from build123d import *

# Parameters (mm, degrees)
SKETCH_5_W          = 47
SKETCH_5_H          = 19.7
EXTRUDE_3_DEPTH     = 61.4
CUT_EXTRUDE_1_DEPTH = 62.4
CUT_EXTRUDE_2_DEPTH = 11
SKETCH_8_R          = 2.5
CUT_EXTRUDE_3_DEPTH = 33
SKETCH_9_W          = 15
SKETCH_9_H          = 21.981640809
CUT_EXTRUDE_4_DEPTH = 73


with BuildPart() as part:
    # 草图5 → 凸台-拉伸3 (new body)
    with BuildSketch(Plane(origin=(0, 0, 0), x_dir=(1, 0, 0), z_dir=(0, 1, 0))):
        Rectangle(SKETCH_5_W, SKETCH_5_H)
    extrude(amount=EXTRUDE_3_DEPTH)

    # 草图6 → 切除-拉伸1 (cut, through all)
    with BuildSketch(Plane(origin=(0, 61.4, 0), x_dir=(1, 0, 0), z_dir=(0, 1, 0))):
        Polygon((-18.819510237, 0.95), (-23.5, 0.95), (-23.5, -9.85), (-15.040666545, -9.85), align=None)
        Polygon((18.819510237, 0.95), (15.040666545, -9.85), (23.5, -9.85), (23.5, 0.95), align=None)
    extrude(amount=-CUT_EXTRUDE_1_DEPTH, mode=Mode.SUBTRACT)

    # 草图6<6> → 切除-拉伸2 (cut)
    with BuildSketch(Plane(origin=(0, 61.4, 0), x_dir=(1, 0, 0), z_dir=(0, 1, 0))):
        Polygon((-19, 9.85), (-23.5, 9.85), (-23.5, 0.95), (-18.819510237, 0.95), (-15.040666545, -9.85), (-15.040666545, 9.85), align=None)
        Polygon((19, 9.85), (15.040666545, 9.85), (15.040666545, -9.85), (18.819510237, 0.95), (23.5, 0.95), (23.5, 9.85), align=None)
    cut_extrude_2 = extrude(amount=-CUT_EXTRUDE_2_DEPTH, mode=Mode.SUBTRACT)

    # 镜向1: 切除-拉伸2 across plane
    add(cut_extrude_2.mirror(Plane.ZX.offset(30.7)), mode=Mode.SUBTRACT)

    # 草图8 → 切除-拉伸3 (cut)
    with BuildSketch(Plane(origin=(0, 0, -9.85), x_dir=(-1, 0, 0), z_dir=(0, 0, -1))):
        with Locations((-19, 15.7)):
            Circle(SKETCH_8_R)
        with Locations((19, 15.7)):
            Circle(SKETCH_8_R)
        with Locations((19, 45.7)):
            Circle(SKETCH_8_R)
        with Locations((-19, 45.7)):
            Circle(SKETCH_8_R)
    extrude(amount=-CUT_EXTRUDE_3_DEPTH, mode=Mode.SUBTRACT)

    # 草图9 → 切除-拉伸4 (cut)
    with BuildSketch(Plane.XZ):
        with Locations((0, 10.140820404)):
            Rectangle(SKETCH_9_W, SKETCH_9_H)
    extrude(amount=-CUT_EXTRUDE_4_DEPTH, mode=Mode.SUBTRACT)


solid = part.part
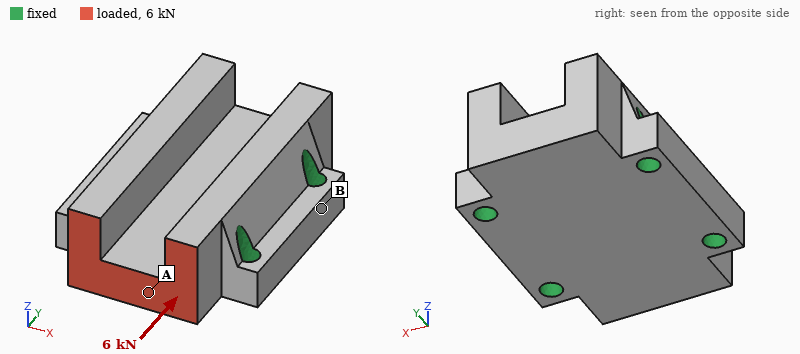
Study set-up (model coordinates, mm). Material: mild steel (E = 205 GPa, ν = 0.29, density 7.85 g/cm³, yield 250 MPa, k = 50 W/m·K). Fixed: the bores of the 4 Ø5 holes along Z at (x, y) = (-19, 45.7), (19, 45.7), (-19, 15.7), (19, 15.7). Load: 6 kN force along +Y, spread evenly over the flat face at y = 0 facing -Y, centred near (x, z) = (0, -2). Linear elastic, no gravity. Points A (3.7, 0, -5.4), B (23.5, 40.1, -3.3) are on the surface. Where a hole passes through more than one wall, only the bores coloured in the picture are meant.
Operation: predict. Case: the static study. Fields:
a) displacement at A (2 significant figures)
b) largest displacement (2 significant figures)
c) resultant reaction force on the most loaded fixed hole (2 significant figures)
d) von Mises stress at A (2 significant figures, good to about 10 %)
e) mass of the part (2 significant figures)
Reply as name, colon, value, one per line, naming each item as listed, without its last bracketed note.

displacement at A: 1.9 µm
largest displacement: 2.3 µm
resultant reaction force on the most loaded fixed hole: 2.1 kN
von Mises stress at A: 11 MPa
mass of the part: 260 g
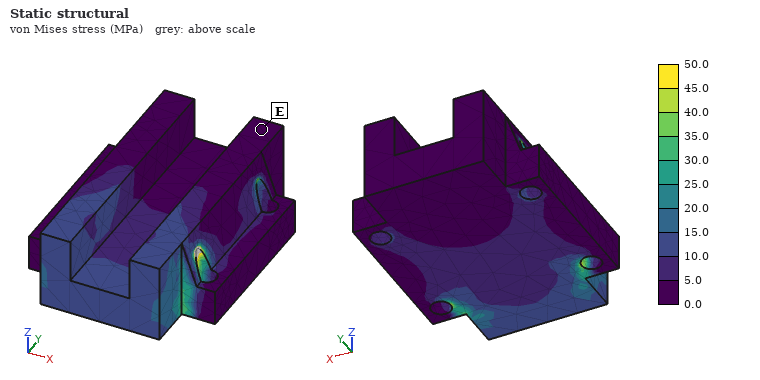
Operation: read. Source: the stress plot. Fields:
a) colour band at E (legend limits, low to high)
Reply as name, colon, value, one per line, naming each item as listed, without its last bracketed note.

colour band at E: 0.0 to 5.0 MPa
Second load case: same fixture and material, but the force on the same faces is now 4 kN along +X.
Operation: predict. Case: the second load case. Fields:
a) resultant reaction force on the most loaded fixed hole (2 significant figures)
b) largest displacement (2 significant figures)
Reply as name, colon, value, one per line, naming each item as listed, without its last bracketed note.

resultant reaction force on the most loaded fixed hole: 2.6 kN
largest displacement: 7.9 µm
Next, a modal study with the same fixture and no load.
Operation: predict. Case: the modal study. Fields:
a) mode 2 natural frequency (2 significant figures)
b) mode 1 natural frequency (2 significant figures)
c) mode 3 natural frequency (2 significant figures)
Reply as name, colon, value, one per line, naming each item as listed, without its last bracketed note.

mode 2 natural frequency: 21 kHz
mode 1 natural frequency: 21 kHz
mode 3 natural frequency: 27 kHz
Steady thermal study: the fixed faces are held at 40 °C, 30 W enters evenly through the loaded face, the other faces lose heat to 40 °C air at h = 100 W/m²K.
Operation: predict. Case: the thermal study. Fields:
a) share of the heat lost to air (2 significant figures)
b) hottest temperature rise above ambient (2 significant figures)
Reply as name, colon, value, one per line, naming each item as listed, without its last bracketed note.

share of the heat lost to air: 14 %
hottest temperature rise above ambient: 27 K
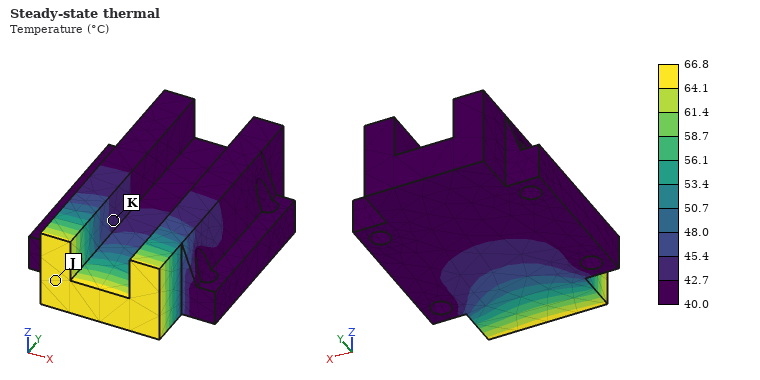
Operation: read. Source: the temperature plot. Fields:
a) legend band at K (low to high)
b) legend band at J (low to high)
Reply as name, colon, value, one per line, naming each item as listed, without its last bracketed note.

legend band at K: 42.7 to 45.4 °C
legend band at J: 64.1 to 66.8 °C
